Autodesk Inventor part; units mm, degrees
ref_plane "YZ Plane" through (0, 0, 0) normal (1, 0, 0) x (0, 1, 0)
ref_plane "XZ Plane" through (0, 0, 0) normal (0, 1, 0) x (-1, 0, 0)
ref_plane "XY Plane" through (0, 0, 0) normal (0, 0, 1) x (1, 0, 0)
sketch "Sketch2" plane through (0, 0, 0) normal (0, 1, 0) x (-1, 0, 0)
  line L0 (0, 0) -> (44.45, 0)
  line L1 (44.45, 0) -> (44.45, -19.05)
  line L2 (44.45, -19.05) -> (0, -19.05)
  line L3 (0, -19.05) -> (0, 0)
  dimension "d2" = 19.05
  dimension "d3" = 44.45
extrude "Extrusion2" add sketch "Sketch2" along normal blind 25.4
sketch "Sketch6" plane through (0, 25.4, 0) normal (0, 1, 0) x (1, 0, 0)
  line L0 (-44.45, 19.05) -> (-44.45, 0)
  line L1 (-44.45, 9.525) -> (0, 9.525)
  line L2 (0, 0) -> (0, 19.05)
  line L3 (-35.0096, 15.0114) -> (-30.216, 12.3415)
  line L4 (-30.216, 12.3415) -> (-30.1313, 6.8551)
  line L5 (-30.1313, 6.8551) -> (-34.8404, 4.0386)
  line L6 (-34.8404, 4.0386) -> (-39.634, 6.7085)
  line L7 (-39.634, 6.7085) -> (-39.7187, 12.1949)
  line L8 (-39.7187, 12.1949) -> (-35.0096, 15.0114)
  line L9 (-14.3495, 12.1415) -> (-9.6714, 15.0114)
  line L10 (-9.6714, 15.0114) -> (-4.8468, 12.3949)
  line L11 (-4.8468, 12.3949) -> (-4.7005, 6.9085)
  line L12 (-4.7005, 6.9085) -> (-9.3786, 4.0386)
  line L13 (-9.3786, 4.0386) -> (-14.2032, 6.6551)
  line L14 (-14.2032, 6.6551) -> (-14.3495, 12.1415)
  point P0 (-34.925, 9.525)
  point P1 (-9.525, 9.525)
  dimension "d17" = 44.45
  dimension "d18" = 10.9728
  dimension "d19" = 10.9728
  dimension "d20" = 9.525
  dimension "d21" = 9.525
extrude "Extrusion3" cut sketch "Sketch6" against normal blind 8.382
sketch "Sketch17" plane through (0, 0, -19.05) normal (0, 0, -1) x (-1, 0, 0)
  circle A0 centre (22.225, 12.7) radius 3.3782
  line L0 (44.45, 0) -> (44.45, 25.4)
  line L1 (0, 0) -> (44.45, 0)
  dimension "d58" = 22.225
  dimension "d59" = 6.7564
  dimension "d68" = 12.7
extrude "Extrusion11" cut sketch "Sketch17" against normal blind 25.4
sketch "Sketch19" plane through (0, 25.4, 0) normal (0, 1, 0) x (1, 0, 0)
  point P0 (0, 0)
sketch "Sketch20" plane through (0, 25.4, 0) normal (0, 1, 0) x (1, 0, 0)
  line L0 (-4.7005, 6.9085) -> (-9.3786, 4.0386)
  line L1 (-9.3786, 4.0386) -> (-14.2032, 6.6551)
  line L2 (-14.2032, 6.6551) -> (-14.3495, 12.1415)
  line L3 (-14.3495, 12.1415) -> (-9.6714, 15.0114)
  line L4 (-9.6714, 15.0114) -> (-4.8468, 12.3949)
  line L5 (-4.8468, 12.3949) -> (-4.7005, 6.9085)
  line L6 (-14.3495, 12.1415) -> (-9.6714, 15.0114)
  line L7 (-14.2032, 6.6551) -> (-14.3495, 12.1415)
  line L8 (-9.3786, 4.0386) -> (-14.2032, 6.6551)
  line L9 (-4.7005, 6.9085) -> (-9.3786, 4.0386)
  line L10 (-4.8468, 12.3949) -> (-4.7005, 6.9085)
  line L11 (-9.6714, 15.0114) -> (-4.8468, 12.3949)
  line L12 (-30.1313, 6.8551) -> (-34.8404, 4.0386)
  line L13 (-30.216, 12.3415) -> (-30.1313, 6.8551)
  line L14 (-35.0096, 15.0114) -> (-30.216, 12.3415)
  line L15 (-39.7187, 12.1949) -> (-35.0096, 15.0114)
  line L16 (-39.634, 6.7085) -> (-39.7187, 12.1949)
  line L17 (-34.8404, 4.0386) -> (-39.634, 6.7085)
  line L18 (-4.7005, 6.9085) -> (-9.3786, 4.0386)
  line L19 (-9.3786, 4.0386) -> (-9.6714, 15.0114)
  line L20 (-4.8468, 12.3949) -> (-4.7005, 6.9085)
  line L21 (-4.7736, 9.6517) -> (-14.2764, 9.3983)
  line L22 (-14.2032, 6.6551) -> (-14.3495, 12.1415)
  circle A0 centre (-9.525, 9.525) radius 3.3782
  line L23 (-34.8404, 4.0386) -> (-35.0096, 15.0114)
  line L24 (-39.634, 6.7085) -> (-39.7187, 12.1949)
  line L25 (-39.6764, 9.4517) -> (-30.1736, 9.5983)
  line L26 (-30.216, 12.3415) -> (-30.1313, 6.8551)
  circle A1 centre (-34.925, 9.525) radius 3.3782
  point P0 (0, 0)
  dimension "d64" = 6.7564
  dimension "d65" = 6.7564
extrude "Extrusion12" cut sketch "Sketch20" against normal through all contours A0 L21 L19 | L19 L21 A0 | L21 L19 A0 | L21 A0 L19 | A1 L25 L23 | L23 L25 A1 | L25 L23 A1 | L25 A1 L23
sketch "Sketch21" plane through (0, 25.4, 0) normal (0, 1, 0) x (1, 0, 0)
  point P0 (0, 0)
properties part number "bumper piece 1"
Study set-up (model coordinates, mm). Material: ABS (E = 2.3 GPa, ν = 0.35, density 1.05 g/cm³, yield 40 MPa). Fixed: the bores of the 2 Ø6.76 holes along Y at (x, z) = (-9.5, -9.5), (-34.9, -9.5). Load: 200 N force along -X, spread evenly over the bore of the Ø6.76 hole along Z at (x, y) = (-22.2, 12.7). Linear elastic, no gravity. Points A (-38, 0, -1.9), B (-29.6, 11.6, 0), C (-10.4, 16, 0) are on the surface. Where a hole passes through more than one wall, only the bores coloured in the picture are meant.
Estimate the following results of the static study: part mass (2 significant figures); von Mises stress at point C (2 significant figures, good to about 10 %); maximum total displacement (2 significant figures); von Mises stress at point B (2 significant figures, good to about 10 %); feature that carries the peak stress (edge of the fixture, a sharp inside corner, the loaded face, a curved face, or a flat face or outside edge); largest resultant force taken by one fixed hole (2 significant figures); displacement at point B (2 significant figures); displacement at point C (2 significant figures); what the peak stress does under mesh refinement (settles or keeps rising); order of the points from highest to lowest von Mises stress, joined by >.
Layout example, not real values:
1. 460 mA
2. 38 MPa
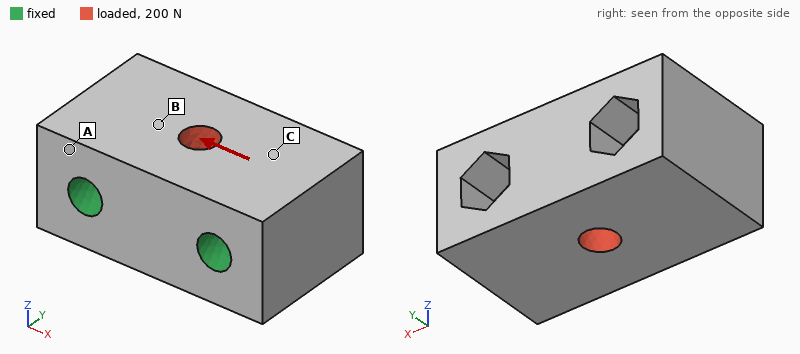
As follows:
1. 19 g
2. 0.19 MPa
3. 2.6 µm
4. 0.38 MPa
5. edge of the fixture
6. 100 N
7. 1.5 µm
8. 1.2 µm
9. keeps rising
10. B > C > A
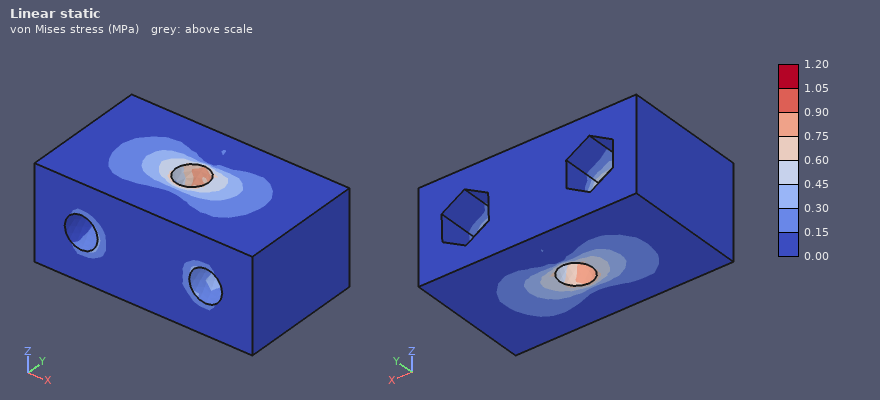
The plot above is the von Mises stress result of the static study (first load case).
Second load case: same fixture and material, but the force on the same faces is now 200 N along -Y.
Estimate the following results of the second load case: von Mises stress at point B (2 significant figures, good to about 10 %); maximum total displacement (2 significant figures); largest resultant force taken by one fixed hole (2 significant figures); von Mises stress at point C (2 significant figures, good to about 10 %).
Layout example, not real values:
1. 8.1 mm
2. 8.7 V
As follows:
1. 0.34 MPa
2. 4.3 µm
3. 100 N
4. 0.20 MPa
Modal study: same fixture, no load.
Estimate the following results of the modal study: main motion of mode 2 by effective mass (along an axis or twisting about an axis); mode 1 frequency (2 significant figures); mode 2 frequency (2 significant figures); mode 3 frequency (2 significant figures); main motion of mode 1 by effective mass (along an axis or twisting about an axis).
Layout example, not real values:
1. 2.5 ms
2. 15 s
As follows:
1. twisting about Y
2. 9000 Hz
3. 11 kHz
4. 12 kHz
5. along Z
